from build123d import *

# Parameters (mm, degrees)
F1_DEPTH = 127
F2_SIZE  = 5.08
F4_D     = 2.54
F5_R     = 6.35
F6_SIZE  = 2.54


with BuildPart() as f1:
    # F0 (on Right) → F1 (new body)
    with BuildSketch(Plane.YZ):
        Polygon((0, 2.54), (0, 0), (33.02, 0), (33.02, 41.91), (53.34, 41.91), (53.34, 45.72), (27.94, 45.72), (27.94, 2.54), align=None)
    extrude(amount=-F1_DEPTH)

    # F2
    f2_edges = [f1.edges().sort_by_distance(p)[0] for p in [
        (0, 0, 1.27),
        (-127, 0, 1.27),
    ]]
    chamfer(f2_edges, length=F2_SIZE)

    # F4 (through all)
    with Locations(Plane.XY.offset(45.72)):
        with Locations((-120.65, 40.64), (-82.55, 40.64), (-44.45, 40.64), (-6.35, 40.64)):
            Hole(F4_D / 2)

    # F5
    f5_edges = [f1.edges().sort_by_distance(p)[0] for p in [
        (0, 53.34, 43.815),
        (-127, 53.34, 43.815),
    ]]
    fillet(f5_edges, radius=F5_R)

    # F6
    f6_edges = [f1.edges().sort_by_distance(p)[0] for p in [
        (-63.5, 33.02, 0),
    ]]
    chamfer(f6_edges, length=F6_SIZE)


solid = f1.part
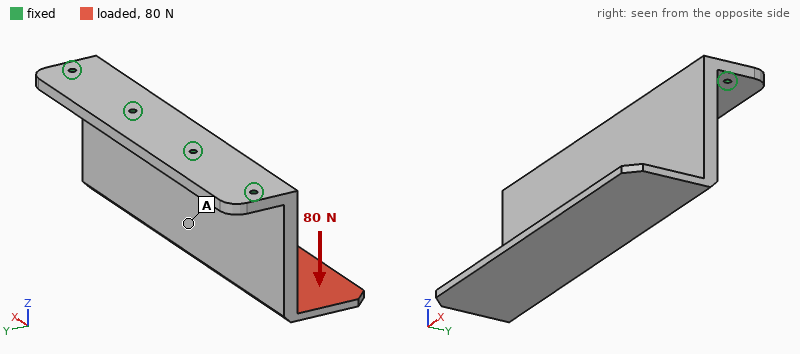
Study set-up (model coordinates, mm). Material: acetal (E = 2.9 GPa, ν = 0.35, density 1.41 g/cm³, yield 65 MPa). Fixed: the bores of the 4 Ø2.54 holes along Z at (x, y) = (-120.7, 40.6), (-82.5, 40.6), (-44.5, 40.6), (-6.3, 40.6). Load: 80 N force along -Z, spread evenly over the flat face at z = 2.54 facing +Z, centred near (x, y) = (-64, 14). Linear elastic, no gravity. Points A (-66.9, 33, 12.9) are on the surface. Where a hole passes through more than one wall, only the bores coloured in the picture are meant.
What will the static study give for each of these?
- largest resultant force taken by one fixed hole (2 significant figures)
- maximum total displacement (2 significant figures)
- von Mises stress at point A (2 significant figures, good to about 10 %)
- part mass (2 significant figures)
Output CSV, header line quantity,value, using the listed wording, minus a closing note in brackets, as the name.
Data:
quantity,value
largest resultant force taken by one fixed hole,26 N
maximum total displacement,1.6 mm
von Mises stress at point A,2.1 MPa
part mass,67 g
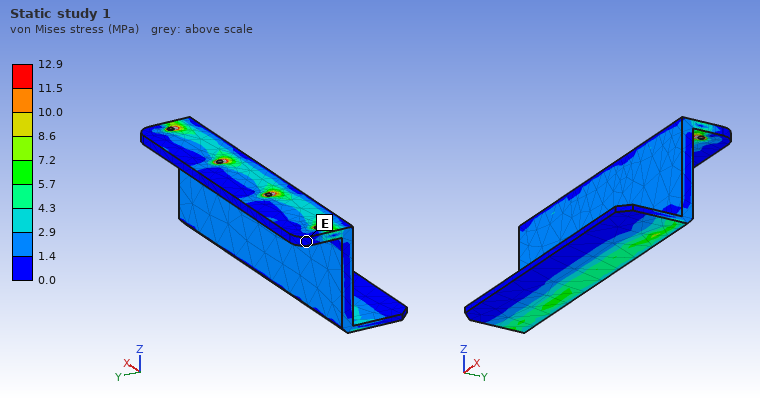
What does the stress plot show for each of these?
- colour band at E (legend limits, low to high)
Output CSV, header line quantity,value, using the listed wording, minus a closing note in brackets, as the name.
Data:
quantity,value
colour band at E,0.0 to 1.4 MPa
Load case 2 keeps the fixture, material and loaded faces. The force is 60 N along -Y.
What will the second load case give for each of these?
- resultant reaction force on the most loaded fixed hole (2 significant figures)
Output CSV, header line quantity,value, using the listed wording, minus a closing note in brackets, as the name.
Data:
quantity,value
resultant reaction force on the most loaded fixed hole,27 N
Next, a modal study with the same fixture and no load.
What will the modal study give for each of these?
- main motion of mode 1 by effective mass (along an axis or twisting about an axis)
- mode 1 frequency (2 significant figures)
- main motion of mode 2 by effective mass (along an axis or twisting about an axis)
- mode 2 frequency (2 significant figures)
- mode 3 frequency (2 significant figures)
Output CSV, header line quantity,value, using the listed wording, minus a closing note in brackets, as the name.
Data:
quantity,value
main motion of mode 1 by effective mass,along Y
mode 1 frequency,210 Hz
main motion of mode 2 by effective mass,twisting about Z
mode 2 frequency,370 Hz
mode 3 frequency,730 Hz
